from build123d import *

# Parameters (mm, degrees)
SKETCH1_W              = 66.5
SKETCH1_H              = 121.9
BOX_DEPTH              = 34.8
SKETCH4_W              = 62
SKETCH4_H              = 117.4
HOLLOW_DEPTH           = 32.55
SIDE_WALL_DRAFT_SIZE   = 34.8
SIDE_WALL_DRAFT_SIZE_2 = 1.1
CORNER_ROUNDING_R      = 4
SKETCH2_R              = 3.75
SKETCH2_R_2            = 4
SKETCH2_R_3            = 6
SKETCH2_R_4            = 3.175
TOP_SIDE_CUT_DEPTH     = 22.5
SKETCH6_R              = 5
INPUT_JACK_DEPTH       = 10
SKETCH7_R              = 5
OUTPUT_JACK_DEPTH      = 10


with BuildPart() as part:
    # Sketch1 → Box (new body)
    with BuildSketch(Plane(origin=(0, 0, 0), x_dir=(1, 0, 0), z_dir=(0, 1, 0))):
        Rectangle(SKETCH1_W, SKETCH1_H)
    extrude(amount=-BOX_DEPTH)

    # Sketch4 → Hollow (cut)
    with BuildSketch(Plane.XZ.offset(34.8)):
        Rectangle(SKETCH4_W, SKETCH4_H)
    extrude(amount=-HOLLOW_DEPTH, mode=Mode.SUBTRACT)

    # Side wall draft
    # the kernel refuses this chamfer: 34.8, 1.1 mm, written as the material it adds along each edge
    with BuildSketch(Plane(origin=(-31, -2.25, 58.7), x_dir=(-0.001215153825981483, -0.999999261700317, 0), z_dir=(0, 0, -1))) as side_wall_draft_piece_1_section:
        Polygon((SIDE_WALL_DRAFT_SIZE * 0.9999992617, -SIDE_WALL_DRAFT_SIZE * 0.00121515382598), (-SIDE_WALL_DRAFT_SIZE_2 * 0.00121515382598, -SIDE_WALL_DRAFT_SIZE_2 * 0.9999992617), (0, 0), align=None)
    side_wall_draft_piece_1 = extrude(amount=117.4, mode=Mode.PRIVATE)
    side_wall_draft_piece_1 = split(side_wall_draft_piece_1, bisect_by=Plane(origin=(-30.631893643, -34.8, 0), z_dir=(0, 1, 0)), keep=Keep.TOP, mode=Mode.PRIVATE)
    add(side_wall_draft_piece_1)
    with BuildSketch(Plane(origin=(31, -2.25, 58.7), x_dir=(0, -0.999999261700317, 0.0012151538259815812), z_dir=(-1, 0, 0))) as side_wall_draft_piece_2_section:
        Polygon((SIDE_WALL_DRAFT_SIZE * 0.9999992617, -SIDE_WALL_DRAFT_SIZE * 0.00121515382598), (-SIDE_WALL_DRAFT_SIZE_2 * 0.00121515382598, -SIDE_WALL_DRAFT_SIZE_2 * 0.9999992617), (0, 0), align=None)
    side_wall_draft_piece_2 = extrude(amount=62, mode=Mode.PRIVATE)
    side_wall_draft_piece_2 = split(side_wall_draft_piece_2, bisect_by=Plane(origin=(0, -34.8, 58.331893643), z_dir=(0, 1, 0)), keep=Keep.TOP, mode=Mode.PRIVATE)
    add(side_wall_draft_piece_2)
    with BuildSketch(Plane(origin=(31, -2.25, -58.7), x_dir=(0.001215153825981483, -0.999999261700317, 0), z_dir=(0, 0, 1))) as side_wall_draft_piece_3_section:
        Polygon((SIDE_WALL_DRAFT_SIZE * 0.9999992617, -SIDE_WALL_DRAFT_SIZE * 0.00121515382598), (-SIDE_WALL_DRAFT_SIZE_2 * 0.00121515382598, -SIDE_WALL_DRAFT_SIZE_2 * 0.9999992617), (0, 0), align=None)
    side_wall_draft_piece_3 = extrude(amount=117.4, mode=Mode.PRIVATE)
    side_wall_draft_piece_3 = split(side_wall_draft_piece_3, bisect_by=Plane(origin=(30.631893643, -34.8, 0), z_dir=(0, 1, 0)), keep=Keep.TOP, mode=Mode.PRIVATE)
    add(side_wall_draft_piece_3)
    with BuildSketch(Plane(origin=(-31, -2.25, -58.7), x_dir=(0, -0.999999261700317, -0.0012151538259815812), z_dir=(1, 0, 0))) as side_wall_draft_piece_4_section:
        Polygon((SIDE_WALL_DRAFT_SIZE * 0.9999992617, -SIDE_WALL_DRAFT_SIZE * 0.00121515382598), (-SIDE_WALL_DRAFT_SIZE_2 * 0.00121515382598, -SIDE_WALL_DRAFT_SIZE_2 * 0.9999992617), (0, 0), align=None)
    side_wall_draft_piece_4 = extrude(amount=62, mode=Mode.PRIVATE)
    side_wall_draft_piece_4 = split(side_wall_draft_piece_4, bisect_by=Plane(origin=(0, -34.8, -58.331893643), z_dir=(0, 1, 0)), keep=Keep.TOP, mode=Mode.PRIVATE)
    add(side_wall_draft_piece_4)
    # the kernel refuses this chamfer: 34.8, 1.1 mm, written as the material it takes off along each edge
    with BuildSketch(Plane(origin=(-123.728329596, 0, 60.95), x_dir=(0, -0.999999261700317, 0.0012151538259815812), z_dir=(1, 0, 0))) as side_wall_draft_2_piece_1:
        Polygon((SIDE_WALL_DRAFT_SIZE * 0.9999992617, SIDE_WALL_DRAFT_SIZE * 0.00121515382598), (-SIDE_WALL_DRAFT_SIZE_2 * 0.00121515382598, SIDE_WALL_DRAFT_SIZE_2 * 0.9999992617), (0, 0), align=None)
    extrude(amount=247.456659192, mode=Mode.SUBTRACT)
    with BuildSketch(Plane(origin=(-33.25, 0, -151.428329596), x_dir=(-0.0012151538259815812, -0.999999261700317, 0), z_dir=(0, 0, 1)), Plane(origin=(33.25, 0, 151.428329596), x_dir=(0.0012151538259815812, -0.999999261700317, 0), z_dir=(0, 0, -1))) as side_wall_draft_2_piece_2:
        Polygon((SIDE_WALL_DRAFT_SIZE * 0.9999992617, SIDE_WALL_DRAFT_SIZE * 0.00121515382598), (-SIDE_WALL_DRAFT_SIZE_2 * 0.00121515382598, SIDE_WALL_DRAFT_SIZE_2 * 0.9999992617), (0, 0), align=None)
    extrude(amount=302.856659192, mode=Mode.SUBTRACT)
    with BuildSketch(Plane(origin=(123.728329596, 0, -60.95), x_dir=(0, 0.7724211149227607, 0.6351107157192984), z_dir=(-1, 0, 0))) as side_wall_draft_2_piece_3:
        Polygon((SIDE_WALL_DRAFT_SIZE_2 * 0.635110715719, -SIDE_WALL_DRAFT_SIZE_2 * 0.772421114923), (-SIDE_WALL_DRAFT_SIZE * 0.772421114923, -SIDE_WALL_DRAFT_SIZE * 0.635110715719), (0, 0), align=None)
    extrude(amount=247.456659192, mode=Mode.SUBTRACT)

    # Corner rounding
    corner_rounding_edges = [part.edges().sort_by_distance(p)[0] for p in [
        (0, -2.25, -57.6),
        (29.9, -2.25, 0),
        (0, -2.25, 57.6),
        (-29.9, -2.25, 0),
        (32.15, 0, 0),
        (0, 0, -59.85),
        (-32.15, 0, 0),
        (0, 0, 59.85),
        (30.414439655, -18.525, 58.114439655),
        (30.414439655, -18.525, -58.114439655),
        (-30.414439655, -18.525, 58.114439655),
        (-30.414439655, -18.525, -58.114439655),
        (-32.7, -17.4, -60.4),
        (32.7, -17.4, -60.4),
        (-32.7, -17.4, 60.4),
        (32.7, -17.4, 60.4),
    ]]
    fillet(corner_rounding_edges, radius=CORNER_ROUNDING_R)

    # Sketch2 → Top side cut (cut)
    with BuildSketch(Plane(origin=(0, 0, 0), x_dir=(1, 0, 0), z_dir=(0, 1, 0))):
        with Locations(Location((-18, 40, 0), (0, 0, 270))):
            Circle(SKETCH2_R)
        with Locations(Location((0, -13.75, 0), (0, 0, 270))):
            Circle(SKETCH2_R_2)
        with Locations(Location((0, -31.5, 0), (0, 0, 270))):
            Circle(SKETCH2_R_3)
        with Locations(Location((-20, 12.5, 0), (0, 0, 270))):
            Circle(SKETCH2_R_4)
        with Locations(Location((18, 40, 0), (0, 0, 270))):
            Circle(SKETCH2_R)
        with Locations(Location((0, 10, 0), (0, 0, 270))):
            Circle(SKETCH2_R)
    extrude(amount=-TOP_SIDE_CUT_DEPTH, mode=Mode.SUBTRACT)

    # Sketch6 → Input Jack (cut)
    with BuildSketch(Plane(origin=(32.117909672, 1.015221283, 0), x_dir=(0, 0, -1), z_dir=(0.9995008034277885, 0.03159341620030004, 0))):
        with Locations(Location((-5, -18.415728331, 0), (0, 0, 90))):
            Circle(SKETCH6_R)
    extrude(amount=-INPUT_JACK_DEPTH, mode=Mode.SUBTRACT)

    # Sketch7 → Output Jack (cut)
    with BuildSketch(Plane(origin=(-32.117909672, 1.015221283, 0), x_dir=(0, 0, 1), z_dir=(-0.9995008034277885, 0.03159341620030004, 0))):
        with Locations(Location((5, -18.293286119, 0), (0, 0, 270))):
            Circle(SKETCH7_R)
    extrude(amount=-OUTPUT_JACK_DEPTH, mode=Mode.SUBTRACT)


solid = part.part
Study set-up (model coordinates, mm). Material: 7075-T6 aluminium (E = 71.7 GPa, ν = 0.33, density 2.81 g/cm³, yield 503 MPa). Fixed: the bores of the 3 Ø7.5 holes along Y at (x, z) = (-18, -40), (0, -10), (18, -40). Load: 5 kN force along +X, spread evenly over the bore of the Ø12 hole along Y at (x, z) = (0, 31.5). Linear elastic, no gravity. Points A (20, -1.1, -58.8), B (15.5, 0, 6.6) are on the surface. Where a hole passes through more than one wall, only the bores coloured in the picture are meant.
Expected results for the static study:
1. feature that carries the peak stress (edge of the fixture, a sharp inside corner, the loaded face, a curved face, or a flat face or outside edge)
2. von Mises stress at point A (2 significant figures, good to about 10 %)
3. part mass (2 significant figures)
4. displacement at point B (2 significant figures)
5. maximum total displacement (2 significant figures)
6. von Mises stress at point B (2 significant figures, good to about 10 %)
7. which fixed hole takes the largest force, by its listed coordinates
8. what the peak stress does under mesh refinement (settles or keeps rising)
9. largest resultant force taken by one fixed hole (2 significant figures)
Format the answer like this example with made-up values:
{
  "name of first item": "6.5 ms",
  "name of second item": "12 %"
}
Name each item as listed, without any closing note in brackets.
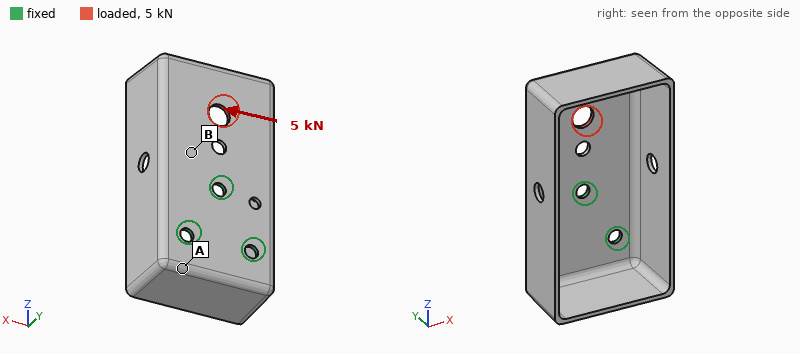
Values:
{
  "feature that carries the peak stress": "edge of the fixture",
  "von Mises stress at point A": "17 MPa",
  "part mass": "120 g",
  "displacement at point B": "0.063 mm",
  "maximum total displacement": "0.30 mm",
  "von Mises stress at point B": "69 MPa",
  "which fixed hole takes the largest force, by its listed coordinates": "(0, -10)",
  "what the peak stress does under mesh refinement": "keeps rising",
  "largest resultant force taken by one fixed hole": "6.8 kN"
}
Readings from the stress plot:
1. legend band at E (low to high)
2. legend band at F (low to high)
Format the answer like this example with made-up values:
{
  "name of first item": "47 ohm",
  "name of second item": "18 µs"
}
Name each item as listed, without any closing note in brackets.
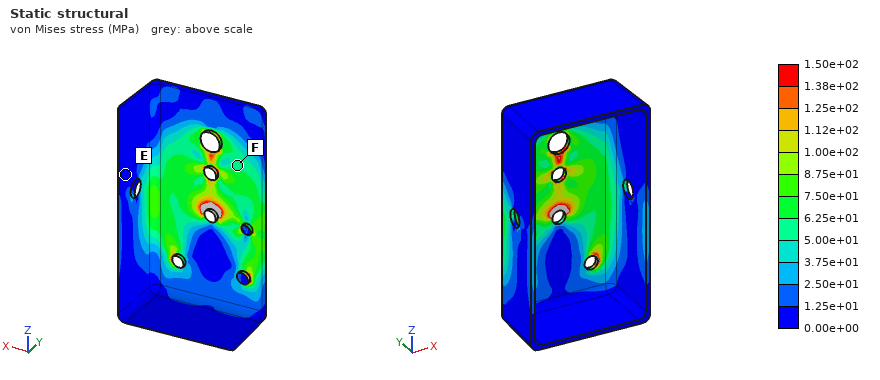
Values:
{
  "legend band at E": "0.00e+00 to 1.25e+01 MPa",
  "legend band at F": "5.00e+01 to 6.25e+01 MPa"
}
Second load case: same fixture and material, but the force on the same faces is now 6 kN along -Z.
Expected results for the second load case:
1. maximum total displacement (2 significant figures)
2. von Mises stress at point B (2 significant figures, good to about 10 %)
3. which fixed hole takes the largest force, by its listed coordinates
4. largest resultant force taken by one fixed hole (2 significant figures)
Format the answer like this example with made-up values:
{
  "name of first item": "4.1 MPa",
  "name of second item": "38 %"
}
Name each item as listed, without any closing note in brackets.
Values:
{
  "maximum total displacement": "57 µm",
  "von Mises stress at point B": "44 MPa",
  "which fixed hole takes the largest force, by its listed coordinates": "(0, -10)",
  "largest resultant force taken by one fixed hole": "3.2 kN"
}
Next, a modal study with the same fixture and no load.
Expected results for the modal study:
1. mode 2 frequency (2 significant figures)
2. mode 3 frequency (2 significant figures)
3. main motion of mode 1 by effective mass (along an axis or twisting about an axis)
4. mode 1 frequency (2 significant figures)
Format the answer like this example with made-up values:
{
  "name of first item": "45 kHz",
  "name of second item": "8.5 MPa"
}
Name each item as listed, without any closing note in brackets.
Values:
{
  "mode 2 frequency": "540 Hz",
  "mode 3 frequency": "1800 Hz",
  "main motion of mode 1 by effective mass": "along Y",
  "mode 1 frequency": "470 Hz"
}
